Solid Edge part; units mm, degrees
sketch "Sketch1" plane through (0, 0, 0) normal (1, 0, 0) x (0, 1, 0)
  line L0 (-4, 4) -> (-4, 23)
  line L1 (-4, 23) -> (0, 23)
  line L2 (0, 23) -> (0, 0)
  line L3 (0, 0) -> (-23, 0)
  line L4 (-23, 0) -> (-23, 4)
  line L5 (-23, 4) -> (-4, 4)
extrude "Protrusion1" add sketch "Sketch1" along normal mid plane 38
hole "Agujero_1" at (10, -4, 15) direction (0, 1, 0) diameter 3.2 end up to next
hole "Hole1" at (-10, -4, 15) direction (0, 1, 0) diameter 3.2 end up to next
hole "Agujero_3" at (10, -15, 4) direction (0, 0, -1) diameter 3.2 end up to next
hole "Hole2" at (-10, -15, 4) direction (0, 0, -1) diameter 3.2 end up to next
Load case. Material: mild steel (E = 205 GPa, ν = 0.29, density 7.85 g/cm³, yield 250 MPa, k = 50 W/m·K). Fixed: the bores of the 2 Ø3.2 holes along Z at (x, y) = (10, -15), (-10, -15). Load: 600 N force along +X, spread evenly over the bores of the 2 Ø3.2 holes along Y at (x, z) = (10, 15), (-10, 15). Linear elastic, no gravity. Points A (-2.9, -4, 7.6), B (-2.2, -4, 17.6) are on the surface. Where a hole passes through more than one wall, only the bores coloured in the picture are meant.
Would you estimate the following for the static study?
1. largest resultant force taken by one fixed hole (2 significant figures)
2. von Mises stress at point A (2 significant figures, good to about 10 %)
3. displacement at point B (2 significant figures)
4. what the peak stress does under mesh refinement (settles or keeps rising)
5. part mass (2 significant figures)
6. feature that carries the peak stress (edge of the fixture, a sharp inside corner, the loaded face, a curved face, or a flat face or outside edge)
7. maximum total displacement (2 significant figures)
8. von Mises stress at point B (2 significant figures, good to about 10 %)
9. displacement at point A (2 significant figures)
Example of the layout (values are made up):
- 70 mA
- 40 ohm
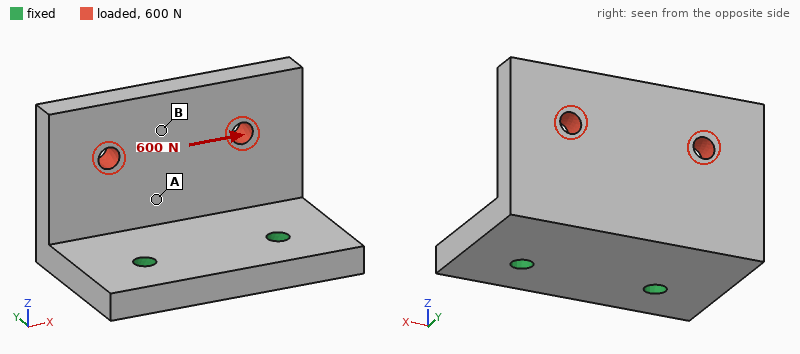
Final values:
- 560 N
- 23 MPa
- 11 µm
- keeps rising
- 49 g
- edge of the fixture
- 18 µm
- 9.1 MPa
- 4.8 µm
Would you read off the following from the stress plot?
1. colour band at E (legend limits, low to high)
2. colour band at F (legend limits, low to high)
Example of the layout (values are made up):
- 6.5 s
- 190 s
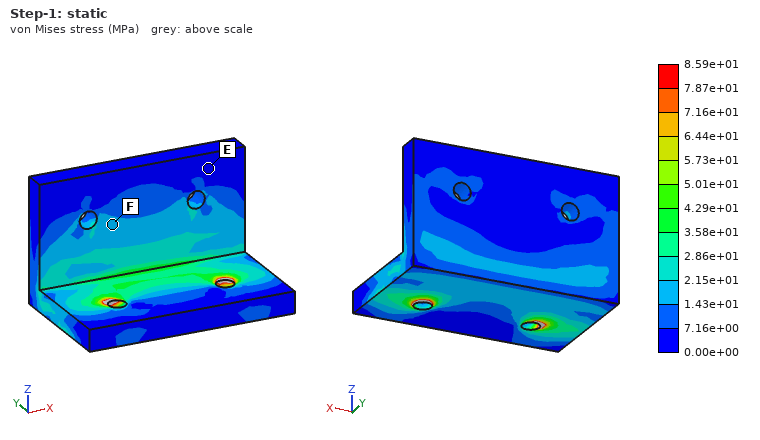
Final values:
- 0.00e+00 to 7.16e+00 MPa
- 1.43e+01 to 2.15e+01 MPa
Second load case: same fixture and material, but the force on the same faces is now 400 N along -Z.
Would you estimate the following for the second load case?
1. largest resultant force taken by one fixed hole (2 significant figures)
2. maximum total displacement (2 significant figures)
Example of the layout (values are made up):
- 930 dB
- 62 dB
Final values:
- 200 N
- 22 µm
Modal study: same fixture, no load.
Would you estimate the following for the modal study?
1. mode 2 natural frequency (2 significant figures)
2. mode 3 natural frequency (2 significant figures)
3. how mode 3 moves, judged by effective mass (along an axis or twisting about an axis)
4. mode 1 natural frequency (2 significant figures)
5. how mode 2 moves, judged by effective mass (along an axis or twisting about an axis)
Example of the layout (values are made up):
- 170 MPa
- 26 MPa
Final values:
- 6400 Hz
- 11 kHz
- along Z
- 3700 Hz
- along X
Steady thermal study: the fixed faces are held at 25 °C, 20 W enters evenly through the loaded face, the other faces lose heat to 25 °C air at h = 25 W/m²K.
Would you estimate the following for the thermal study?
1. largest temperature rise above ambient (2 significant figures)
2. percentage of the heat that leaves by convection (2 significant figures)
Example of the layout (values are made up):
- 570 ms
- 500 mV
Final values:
- 70 K
- 15 %
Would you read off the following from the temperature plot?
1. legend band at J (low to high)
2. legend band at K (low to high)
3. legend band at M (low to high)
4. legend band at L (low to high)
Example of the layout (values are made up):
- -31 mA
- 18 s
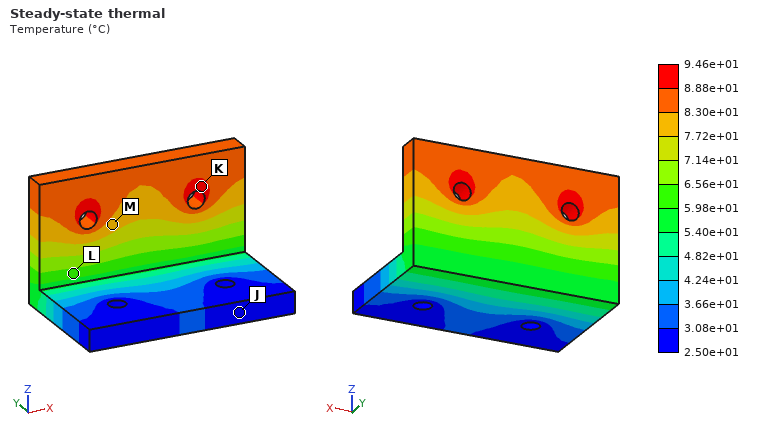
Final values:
- 2.50e+01 to 3.08e+01 °C
- 8.88e+01 to 9.46e+01 °C
- 7.72e+01 to 8.30e+01 °C
- 5.98e+01 to 6.56e+01 °C
